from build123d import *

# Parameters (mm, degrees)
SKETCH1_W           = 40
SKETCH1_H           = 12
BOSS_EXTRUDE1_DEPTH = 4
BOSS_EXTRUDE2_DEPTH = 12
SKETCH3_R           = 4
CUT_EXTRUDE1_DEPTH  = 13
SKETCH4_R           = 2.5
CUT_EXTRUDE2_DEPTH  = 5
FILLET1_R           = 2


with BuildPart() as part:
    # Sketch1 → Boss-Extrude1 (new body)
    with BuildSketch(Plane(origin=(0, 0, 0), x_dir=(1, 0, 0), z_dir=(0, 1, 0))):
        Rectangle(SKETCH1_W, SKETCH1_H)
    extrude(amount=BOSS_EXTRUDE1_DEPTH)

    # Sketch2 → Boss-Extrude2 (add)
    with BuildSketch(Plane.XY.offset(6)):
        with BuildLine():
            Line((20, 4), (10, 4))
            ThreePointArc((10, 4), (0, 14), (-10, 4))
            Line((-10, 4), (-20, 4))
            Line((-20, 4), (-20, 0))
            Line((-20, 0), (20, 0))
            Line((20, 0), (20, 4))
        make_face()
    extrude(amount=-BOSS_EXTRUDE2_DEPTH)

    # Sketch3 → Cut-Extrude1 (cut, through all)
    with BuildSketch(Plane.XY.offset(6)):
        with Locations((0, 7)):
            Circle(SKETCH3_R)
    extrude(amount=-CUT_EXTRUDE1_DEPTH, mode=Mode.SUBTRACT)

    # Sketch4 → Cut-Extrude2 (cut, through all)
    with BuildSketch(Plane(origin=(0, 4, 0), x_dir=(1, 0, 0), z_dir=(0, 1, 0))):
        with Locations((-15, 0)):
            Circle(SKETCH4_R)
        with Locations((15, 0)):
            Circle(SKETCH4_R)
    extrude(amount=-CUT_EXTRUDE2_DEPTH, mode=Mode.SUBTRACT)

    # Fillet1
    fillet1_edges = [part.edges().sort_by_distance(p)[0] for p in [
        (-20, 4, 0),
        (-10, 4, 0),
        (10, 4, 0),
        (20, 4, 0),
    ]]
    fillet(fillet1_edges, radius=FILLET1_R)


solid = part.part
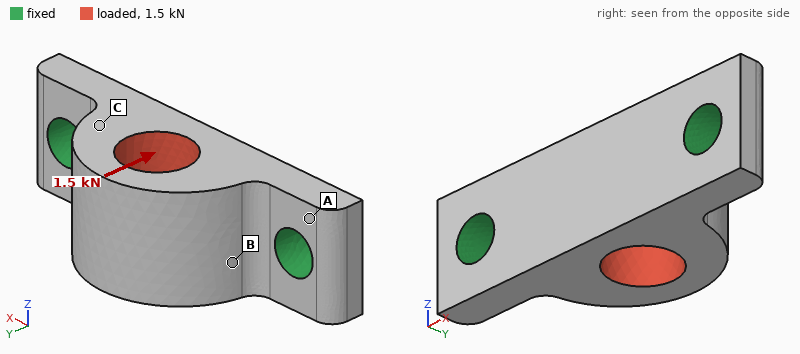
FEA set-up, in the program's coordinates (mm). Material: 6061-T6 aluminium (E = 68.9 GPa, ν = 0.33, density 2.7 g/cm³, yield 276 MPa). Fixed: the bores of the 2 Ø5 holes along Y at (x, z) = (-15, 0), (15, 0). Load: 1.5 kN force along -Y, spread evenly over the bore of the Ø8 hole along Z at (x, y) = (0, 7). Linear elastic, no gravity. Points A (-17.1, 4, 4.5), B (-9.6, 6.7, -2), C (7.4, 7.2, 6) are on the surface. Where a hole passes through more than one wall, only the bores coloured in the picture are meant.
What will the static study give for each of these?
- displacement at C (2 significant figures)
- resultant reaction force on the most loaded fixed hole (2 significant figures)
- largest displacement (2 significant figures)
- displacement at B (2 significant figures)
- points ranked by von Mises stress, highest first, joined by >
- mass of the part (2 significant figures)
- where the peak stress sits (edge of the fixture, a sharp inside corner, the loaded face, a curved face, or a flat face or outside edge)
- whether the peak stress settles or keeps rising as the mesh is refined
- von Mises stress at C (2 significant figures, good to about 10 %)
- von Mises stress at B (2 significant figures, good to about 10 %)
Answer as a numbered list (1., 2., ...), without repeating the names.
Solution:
1. 7.8 µm
2. 820 N
3. 11 µm
4. 6.3 µm
5. B > C > A
6. 8.2 g
7. edge of the fixture
8. keeps rising
9. 18 MPa
10. 29 MPa
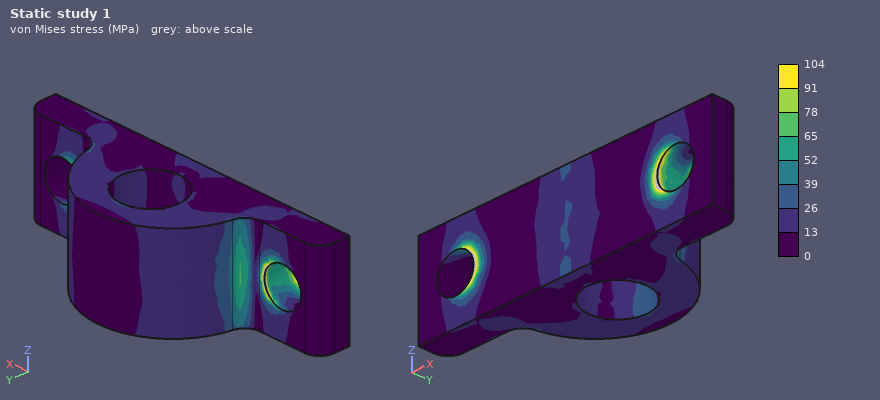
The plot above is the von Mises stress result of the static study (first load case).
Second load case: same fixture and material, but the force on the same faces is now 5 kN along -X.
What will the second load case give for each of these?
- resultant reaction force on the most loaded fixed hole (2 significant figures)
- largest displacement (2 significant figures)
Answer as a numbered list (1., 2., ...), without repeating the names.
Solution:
1. 2.7 kN
2. 20 µm
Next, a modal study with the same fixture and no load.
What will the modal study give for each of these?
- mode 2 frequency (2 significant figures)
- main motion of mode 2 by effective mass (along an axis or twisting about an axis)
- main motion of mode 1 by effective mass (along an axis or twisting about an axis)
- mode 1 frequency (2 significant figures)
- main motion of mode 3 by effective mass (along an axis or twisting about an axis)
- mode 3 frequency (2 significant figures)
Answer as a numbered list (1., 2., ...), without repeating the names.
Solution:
1. 28 kHz
2. along Y
3. along Z
4. 16 kHz
5. along Z
6. 37 kHz
